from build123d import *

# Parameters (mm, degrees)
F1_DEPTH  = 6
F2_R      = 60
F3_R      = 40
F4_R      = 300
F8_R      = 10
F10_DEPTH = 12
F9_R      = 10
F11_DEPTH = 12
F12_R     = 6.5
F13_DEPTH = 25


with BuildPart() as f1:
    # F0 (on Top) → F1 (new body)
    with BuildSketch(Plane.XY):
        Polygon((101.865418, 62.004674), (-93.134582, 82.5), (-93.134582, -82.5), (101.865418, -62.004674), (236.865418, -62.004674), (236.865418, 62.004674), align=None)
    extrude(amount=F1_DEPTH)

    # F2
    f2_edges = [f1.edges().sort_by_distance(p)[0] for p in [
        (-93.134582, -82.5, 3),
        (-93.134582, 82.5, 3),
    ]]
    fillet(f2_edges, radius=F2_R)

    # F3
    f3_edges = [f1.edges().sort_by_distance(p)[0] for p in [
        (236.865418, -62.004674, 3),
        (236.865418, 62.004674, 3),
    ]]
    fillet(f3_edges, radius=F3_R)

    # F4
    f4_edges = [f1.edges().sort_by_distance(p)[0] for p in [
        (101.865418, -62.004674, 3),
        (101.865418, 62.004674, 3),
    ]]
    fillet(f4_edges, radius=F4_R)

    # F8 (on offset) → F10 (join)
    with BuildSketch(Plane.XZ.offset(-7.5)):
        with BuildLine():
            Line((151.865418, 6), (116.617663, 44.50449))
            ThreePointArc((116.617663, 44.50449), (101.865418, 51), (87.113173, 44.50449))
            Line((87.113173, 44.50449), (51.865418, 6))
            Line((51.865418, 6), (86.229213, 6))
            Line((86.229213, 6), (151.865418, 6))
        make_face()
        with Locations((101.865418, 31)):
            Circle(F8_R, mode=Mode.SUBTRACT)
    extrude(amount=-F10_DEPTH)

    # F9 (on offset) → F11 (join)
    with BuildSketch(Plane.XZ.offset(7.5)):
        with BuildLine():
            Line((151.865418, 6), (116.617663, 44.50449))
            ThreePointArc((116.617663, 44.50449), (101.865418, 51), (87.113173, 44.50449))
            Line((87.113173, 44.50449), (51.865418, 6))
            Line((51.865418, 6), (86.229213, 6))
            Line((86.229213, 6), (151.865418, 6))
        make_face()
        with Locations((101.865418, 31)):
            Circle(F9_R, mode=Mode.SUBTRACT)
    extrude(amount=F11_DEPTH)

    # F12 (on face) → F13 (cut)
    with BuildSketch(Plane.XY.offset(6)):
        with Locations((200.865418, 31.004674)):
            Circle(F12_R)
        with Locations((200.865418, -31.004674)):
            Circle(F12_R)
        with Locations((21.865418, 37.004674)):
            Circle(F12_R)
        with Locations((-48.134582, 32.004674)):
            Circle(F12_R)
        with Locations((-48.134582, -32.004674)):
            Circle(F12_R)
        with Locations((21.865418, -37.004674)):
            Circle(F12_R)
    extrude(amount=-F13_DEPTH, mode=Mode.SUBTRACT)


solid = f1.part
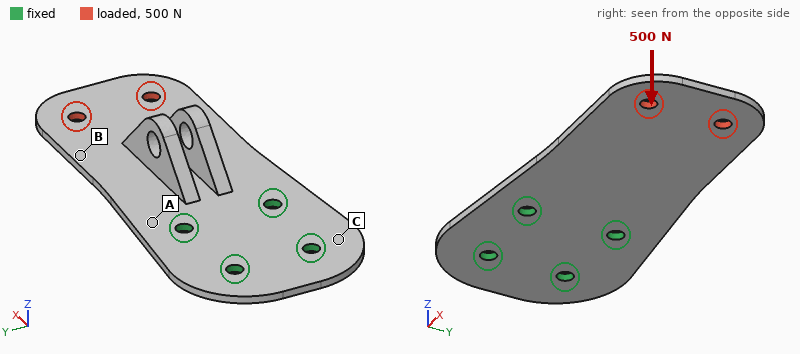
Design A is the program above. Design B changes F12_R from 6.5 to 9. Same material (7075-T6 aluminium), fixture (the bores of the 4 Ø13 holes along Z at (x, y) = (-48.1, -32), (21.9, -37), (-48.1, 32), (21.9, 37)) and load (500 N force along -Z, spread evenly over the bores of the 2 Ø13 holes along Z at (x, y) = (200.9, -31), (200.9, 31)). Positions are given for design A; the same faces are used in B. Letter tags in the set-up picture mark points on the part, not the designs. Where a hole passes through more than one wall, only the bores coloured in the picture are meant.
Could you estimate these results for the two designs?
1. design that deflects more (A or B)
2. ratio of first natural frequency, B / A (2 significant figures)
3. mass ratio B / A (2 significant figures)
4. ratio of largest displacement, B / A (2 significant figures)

A
1.1
0.99
0.92
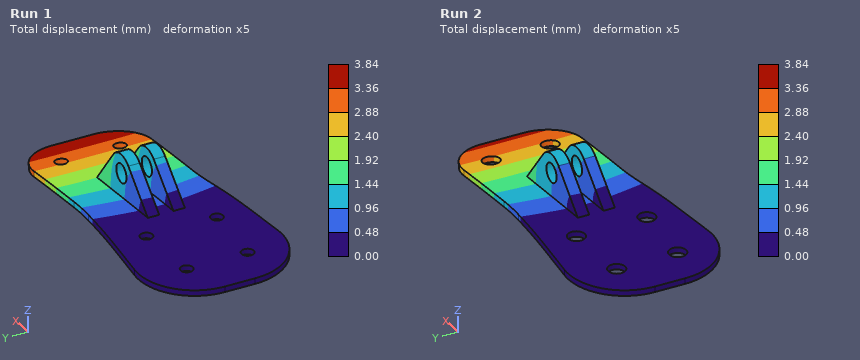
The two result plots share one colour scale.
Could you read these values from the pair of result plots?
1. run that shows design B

Run 2
